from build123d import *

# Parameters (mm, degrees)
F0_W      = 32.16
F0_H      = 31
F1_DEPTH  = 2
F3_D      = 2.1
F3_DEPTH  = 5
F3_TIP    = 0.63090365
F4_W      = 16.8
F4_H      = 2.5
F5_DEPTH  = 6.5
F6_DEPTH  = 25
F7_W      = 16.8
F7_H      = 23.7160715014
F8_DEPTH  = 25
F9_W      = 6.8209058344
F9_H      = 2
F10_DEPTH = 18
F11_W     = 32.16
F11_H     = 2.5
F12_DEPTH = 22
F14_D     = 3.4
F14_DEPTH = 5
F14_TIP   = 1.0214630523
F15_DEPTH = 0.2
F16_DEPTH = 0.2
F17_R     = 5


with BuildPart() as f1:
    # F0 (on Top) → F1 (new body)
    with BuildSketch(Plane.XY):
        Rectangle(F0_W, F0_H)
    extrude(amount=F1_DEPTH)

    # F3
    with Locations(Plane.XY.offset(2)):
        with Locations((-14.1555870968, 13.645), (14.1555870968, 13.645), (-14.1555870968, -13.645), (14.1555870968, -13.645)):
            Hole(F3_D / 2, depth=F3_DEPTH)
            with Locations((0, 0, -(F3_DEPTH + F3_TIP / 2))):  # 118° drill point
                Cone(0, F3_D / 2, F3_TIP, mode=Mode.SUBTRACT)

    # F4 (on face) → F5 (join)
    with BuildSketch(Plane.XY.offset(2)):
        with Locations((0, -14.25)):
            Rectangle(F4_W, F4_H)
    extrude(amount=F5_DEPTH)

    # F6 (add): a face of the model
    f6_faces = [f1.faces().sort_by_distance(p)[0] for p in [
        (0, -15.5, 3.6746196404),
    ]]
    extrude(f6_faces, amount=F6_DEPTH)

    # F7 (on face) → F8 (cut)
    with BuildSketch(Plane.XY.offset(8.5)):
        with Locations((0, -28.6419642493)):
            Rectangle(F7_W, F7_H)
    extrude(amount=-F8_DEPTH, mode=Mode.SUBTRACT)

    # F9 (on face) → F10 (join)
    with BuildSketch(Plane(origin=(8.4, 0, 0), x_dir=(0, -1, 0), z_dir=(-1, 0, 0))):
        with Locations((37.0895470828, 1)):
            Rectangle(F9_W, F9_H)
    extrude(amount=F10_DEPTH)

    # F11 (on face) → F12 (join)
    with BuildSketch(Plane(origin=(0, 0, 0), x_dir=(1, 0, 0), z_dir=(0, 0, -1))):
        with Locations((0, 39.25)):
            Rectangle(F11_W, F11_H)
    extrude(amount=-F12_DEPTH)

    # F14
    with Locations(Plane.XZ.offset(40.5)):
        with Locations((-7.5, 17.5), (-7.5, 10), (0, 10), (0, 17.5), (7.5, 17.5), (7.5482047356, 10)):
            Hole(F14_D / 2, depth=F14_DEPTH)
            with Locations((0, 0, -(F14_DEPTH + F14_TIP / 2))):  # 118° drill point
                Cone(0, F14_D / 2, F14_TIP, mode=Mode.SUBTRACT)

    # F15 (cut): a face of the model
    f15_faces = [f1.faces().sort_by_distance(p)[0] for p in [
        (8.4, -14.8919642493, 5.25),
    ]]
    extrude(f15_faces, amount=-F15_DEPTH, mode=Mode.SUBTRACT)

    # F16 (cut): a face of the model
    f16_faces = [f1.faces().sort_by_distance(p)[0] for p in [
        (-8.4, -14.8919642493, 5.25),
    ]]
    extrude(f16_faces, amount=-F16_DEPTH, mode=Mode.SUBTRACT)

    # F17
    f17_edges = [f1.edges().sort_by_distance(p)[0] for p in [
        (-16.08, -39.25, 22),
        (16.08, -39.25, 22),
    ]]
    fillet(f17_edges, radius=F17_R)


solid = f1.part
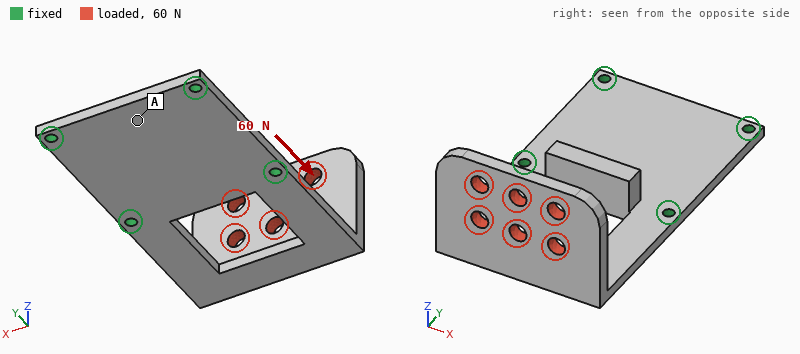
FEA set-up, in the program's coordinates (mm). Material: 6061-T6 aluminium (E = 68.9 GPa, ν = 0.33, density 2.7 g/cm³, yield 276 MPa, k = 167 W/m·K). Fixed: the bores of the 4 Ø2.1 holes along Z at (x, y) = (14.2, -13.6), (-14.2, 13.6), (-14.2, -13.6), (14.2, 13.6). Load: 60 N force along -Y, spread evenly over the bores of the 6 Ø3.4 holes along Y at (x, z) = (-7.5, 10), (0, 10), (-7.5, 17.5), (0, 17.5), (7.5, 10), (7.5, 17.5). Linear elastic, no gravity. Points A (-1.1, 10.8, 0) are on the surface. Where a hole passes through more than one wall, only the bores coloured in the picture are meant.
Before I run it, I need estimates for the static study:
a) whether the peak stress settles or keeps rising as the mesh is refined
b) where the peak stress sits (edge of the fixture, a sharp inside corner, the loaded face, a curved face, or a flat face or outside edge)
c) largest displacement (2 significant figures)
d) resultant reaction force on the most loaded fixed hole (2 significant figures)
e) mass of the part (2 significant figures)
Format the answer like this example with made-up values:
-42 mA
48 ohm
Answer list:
keeps rising
a sharp inside corner
0.67 mm
29 N
13 g
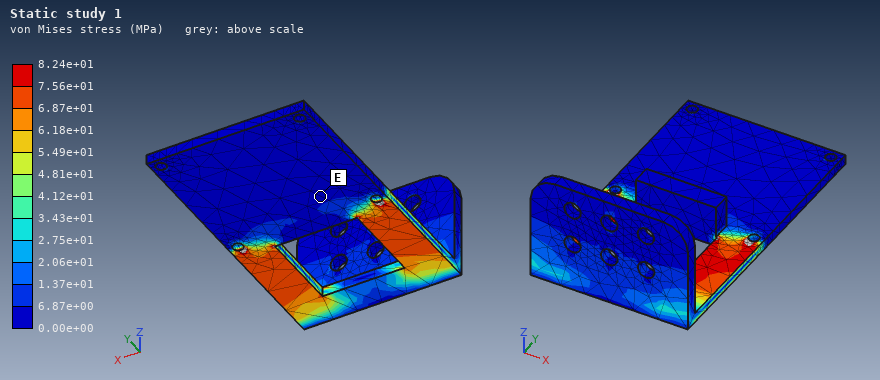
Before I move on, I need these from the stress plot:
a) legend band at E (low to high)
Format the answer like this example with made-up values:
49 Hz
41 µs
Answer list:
0.00e+00 to 6.87e+00 MPa
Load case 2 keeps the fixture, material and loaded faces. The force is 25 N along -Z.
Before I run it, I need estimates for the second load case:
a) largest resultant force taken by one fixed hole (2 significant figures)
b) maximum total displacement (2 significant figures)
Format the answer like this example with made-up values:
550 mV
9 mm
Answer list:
15 N
0.30 mm
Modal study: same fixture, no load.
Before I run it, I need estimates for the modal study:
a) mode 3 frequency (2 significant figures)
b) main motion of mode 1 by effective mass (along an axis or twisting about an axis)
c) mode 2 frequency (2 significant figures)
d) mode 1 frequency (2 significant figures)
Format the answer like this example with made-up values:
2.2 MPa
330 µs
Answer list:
2600 Hz
along Z
1600 Hz
690 Hz
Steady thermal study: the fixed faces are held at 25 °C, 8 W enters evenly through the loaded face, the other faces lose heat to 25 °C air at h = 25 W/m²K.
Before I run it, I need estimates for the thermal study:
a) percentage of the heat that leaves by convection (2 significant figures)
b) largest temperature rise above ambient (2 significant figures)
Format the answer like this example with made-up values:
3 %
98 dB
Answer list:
23 %
39 K
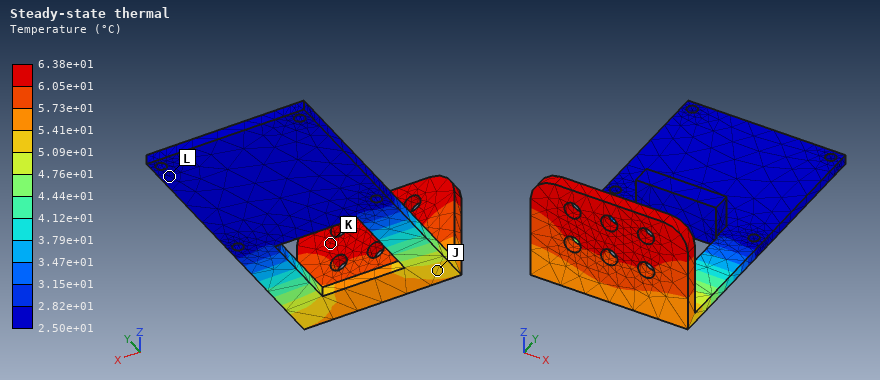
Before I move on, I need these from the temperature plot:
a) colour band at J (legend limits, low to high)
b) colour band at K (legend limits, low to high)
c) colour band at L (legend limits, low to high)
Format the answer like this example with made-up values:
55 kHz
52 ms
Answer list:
5.09e+01 to 5.41e+01 °C
6.05e+01 to 6.38e+01 °C
2.50e+01 to 2.82e+01 °C
